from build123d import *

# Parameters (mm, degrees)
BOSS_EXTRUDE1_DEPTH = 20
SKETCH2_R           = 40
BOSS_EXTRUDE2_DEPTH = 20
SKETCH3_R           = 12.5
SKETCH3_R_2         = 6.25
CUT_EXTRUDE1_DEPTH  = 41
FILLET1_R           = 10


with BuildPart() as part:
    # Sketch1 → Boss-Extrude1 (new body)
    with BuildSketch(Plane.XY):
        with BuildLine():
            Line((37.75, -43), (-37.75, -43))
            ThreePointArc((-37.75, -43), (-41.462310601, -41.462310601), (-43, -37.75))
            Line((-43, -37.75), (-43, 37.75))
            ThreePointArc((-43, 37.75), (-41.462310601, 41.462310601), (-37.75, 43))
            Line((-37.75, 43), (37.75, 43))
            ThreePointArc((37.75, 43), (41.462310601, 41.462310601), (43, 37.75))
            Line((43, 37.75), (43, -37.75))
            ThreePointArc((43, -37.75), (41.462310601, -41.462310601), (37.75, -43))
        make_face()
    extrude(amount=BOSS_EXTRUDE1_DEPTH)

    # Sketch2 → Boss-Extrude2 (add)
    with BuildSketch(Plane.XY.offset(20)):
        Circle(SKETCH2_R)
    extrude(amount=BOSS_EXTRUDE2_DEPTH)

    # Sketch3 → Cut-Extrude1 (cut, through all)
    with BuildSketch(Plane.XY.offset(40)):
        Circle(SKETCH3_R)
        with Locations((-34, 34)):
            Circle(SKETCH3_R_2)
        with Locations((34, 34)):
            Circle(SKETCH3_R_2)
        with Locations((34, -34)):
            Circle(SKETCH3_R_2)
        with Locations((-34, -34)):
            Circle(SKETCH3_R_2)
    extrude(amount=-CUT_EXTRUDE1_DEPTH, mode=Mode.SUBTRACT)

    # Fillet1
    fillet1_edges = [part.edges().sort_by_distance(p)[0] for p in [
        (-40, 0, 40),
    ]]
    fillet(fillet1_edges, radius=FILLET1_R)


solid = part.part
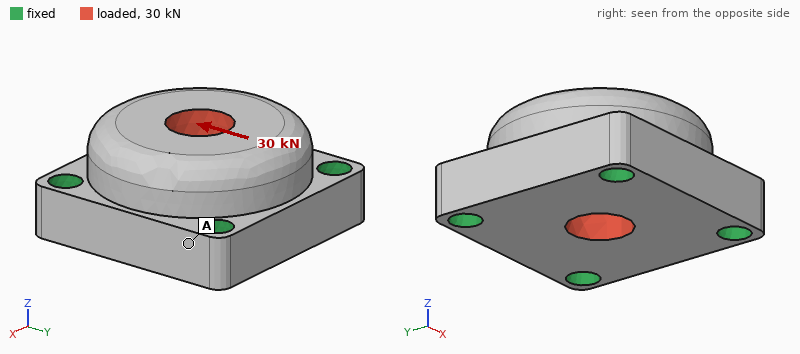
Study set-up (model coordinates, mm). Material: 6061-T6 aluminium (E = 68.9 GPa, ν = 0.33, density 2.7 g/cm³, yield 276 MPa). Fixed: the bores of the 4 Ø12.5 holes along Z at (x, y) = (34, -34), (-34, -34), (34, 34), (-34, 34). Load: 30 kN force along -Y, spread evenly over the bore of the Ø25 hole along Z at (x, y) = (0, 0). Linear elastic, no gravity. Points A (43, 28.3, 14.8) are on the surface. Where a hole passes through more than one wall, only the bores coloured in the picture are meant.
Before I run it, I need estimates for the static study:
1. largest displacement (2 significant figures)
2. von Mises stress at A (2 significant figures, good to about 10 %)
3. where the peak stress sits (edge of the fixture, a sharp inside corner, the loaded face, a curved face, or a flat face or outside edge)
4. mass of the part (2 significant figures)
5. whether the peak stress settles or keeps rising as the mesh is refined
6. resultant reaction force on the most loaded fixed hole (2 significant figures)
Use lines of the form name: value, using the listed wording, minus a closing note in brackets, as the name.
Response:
largest displacement: 12 µm
von Mises stress at A: 6.7 MPa
where the peak stress sits: edge of the fixture
mass of the part: 580 g
whether the peak stress settles or keeps rising as the mesh is refined: keeps rising
resultant reaction force on the most loaded fixed hole: 8.5 kN
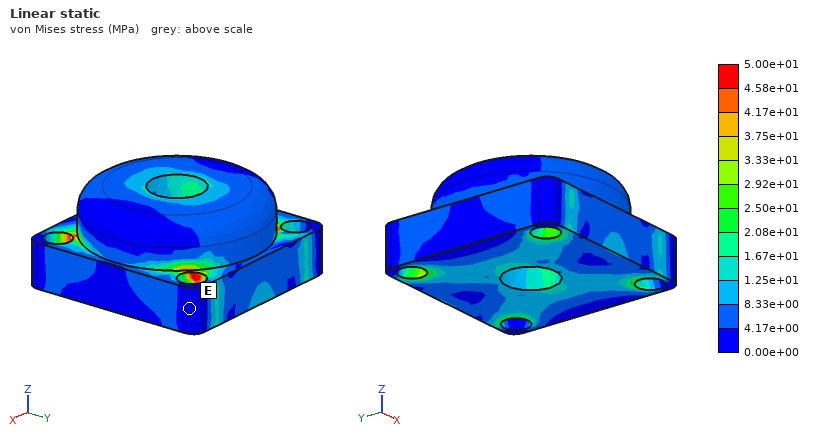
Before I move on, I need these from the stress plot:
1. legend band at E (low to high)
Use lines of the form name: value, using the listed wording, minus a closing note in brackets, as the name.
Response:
legend band at E: 0.00e+00 to 4.17e+00 MPa
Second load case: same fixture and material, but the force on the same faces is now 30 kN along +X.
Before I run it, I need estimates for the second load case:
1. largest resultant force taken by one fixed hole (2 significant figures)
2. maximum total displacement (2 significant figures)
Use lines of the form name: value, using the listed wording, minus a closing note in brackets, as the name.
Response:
largest resultant force taken by one fixed hole: 8.5 kN
maximum total displacement: 12 µm
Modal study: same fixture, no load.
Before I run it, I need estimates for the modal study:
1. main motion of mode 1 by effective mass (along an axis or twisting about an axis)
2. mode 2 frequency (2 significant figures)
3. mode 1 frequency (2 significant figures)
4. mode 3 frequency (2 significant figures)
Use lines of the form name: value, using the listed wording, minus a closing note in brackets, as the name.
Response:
main motion of mode 1 by effective mass: along Z
mode 2 frequency: 15 kHz
mode 1 frequency: 13 kHz
mode 3 frequency: 15 kHz
